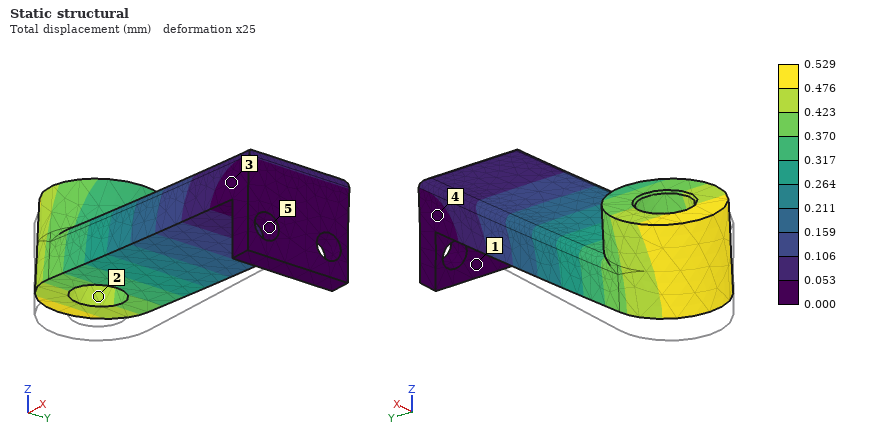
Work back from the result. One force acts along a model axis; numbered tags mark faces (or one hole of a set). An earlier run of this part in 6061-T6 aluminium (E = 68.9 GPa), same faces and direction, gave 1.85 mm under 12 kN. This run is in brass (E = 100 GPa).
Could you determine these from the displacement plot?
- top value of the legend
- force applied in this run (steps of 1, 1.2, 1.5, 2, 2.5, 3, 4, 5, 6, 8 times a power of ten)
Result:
0.529 mm
5 kN
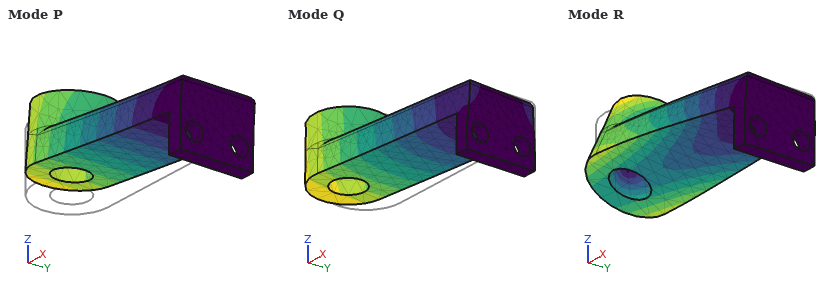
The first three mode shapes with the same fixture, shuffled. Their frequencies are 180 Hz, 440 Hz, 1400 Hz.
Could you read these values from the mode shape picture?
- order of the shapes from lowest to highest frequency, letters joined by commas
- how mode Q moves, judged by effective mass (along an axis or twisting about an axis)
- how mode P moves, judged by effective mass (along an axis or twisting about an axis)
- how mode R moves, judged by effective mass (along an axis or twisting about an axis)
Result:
P, Q, R
along Y
along Z
twisting about X
